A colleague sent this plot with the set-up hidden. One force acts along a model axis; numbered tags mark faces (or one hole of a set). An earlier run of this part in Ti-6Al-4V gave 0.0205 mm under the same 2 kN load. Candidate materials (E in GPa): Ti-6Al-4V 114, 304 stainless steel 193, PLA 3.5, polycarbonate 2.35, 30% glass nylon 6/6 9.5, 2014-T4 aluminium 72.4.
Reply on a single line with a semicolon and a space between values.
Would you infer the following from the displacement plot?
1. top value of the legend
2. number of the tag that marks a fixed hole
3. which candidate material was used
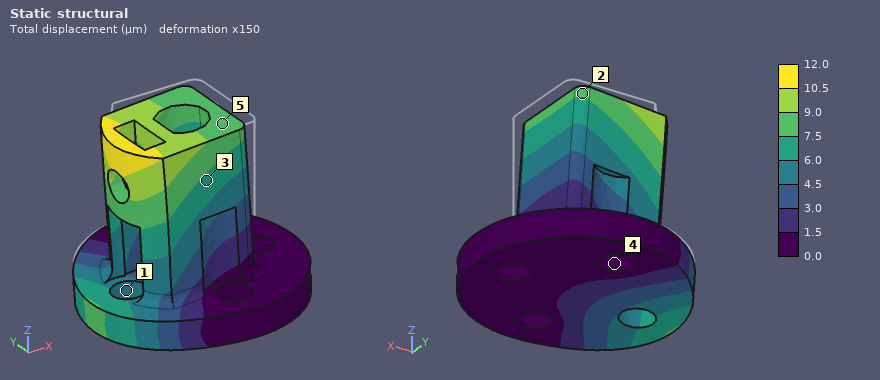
12.0 µm; 4; 304 stainless steel
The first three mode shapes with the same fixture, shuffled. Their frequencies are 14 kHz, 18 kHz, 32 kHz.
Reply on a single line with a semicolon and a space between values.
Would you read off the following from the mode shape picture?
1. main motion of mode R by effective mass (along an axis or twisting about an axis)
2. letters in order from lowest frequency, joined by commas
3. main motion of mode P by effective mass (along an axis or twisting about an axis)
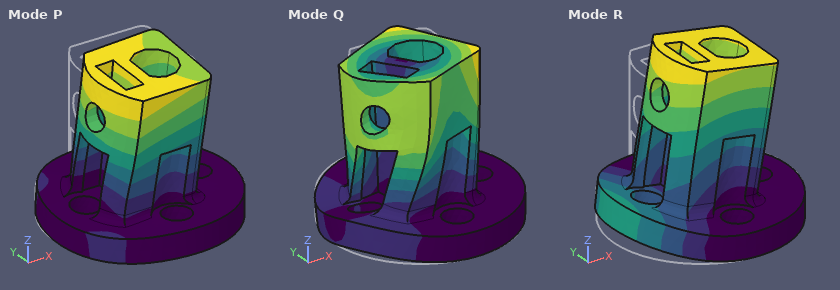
along X; R, P, Q; along Y
